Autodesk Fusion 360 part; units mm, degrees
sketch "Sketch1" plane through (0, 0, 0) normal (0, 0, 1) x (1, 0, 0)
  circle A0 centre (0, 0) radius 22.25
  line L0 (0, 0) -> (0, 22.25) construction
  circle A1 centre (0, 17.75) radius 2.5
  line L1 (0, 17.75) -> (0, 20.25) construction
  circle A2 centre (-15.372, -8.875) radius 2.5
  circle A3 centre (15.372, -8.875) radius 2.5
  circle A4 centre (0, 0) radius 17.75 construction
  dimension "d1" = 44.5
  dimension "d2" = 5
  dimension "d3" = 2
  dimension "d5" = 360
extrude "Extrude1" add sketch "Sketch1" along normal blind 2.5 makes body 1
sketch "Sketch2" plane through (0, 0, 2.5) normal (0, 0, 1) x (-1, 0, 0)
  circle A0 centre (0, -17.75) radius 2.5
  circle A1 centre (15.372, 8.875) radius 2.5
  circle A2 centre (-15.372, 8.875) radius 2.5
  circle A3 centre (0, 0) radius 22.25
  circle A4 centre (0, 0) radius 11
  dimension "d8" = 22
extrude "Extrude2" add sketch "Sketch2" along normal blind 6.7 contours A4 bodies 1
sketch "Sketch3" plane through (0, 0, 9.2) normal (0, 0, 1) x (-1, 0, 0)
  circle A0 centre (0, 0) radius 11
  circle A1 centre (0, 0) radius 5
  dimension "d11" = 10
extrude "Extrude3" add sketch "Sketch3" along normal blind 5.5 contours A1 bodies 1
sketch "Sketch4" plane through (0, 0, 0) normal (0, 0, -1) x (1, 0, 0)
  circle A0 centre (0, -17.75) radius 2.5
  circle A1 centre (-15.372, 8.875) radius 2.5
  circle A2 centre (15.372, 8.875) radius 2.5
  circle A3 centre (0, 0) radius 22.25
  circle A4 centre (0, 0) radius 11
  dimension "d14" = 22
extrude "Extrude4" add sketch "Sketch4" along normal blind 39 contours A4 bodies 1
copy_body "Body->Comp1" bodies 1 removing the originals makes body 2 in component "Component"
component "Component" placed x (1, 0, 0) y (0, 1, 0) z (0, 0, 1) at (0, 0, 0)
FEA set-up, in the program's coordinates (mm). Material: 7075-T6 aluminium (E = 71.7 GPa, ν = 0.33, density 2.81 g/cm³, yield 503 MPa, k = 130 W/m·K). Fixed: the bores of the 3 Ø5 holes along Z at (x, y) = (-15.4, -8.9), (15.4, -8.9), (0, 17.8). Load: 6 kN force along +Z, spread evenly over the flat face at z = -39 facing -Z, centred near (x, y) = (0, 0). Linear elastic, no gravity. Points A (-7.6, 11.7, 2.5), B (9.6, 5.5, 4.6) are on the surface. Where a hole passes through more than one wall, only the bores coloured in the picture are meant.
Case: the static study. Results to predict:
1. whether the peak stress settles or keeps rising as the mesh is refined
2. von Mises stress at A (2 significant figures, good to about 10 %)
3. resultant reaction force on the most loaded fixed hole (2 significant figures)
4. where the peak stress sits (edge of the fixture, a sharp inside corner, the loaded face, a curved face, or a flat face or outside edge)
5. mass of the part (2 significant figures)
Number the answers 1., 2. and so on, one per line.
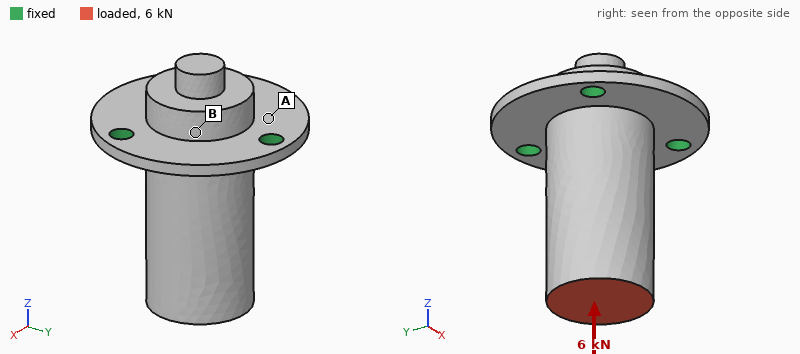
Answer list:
1. keeps rising
2. 72 MPa
3. 2.0 kN
4. edge of the fixture
5. 61 g
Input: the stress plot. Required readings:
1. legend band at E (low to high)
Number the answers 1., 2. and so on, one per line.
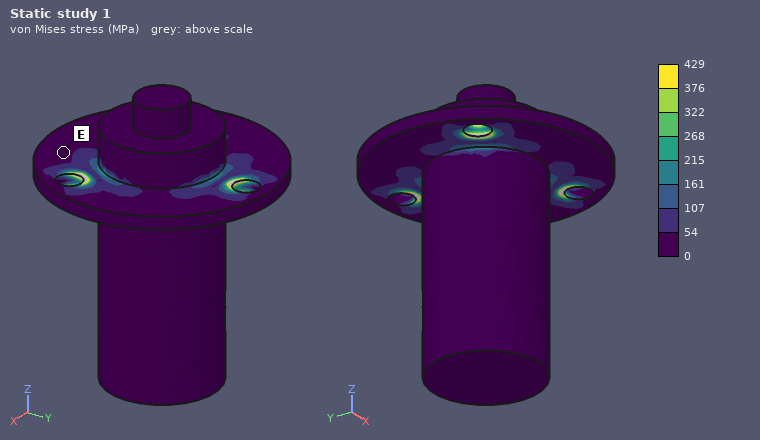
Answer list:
1. 0 to 54 MPa
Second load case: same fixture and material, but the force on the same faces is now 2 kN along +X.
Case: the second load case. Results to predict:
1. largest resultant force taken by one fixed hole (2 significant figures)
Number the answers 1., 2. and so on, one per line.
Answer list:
1. 3.2 kN
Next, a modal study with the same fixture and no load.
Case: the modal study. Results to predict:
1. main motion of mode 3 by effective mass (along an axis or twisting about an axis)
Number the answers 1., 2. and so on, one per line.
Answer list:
1. along Z
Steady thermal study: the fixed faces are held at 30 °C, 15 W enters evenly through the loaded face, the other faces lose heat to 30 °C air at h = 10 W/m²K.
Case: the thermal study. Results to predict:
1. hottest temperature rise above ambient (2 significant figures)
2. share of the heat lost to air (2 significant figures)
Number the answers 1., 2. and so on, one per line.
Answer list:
1. 18 K
2. 3.2 %
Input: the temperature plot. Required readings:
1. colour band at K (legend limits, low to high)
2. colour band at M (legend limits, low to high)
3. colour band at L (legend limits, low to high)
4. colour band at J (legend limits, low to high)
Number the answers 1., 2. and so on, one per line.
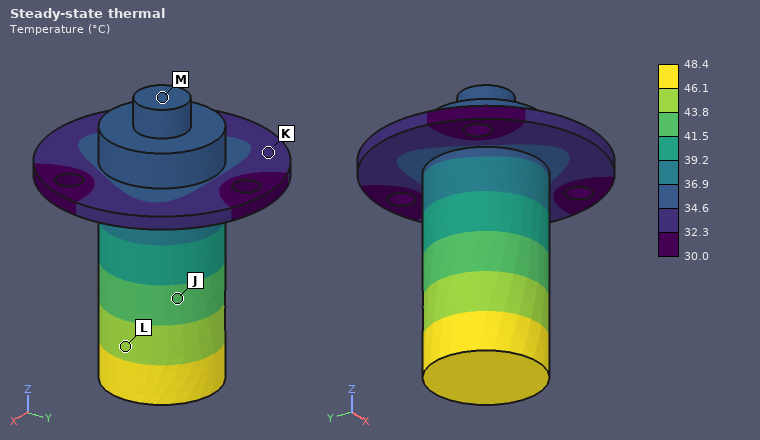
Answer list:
1. 32.3 to 34.6 °C
2. 34.6 to 36.9 °C
3. 43.8 to 46.1 °C
4. 41.5 to 43.8 °C
